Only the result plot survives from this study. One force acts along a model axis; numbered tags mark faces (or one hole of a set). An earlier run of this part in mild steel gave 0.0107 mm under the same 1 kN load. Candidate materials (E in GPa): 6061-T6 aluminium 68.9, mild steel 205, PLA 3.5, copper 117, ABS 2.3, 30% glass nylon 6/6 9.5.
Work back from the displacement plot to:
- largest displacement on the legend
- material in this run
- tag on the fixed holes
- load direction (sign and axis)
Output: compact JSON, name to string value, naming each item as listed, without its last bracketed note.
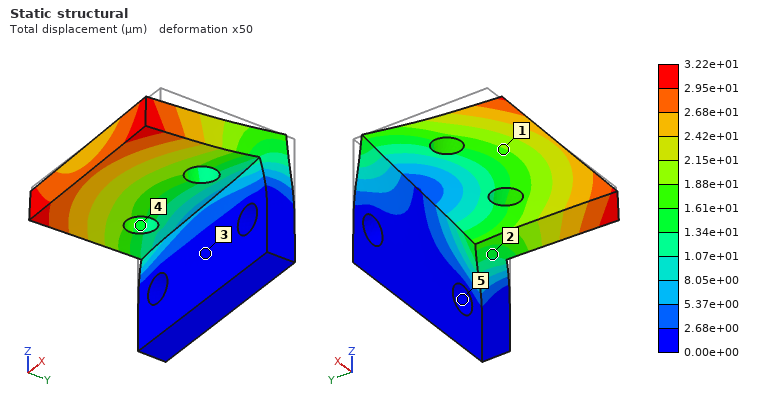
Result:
{"largest displacement on the legend": "3.22e+01 µm", "material in this run": "6061-T6 aluminium", "tag on the fixed holes": "5", "load direction": "-X"}
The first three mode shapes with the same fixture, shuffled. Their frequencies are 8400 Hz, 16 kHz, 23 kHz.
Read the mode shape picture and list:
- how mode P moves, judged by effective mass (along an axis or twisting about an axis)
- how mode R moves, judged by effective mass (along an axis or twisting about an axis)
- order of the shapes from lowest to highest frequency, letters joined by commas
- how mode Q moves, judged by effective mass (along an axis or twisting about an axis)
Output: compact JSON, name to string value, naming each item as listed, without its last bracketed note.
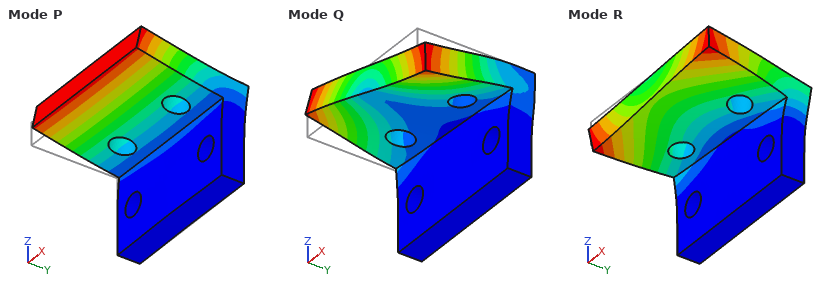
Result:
{"how mode P moves, judged by effective mass": "along Z", "how mode R moves, judged by effective mass": "along X", "order of the shapes from lowest to highest frequency, letters joined by commas": "P, R, Q", "how mode Q moves, judged by effective mass": "along X"}
